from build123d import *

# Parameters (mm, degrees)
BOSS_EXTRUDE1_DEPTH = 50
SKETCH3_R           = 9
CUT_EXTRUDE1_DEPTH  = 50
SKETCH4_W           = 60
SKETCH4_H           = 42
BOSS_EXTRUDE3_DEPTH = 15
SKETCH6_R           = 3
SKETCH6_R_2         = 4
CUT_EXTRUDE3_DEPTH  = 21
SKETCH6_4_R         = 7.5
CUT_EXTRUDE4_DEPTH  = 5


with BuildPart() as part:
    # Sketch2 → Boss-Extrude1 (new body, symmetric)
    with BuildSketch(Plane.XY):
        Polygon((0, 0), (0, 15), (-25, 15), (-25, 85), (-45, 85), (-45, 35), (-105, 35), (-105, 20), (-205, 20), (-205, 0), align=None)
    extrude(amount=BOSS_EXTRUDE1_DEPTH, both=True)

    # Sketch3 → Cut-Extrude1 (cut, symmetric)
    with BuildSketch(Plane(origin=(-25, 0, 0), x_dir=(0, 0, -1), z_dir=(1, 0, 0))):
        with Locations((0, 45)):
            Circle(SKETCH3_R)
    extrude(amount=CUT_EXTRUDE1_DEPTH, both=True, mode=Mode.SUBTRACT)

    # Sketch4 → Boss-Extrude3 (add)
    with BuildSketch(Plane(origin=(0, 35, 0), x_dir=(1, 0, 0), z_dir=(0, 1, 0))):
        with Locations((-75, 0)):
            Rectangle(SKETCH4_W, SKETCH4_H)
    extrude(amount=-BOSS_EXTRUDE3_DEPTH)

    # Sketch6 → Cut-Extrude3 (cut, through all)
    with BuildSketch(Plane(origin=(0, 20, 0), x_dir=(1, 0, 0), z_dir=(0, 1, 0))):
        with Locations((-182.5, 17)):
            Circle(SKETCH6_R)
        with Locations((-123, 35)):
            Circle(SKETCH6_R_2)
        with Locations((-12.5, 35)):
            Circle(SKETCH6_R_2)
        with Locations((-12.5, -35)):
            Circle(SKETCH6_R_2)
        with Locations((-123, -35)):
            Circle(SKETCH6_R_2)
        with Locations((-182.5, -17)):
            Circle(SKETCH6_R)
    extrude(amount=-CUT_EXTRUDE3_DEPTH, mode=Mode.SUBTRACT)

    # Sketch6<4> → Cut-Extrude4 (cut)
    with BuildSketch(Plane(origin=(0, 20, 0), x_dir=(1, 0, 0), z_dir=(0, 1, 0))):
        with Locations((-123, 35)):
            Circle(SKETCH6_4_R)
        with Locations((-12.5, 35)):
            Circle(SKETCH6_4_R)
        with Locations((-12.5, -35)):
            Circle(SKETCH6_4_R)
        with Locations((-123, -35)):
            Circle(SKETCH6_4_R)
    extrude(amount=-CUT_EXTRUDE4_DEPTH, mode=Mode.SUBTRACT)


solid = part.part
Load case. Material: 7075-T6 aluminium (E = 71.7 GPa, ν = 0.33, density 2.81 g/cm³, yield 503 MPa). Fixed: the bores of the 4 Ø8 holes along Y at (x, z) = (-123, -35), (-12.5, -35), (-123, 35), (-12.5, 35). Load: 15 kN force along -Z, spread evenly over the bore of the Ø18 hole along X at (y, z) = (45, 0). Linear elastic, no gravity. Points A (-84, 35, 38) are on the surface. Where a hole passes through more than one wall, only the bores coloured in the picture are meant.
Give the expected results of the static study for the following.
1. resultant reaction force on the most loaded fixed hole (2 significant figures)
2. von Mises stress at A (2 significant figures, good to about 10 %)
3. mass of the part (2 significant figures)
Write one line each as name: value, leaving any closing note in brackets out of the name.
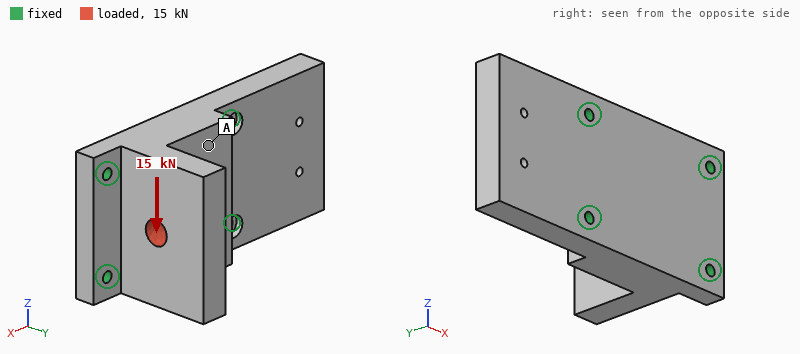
resultant reaction force on the most loaded fixed hole: 7.2 kN
von Mises stress at A: 6.3 MPa
mass of the part: 1.7 kg
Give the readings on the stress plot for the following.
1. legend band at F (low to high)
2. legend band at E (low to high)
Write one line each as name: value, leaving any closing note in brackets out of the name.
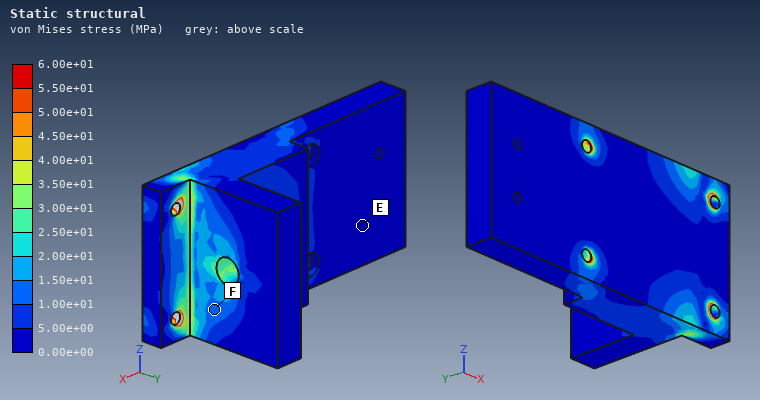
legend band at F: 1.00e+01 to 1.50e+01 MPa
legend band at E: 0.00e+00 to 5.00e+00 MPa
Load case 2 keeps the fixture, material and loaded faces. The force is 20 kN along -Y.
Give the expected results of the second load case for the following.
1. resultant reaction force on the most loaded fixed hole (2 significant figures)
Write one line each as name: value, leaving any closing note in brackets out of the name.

resultant reaction force on the most loaded fixed hole: 8.6 kN
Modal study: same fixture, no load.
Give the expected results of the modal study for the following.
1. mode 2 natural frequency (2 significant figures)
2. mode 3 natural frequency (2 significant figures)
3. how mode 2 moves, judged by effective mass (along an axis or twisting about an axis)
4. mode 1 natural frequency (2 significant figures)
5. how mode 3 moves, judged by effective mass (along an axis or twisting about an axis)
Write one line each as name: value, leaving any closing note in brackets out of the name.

mode 2 natural frequency: 3600 Hz
mode 3 natural frequency: 4100 Hz
how mode 2 moves, judged by effective mass: along X
mode 1 natural frequency: 1900 Hz
how mode 3 moves, judged by effective mass: along Z
